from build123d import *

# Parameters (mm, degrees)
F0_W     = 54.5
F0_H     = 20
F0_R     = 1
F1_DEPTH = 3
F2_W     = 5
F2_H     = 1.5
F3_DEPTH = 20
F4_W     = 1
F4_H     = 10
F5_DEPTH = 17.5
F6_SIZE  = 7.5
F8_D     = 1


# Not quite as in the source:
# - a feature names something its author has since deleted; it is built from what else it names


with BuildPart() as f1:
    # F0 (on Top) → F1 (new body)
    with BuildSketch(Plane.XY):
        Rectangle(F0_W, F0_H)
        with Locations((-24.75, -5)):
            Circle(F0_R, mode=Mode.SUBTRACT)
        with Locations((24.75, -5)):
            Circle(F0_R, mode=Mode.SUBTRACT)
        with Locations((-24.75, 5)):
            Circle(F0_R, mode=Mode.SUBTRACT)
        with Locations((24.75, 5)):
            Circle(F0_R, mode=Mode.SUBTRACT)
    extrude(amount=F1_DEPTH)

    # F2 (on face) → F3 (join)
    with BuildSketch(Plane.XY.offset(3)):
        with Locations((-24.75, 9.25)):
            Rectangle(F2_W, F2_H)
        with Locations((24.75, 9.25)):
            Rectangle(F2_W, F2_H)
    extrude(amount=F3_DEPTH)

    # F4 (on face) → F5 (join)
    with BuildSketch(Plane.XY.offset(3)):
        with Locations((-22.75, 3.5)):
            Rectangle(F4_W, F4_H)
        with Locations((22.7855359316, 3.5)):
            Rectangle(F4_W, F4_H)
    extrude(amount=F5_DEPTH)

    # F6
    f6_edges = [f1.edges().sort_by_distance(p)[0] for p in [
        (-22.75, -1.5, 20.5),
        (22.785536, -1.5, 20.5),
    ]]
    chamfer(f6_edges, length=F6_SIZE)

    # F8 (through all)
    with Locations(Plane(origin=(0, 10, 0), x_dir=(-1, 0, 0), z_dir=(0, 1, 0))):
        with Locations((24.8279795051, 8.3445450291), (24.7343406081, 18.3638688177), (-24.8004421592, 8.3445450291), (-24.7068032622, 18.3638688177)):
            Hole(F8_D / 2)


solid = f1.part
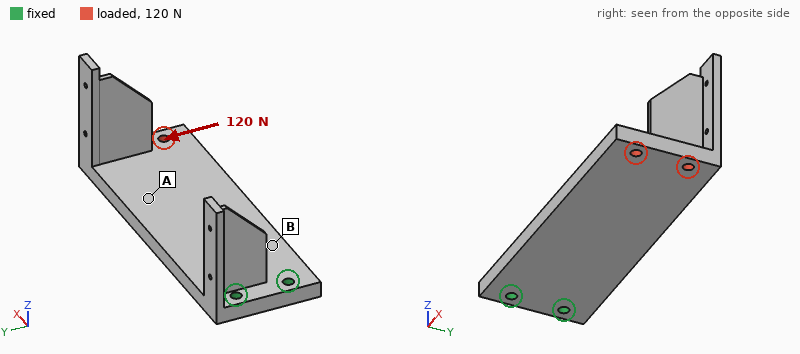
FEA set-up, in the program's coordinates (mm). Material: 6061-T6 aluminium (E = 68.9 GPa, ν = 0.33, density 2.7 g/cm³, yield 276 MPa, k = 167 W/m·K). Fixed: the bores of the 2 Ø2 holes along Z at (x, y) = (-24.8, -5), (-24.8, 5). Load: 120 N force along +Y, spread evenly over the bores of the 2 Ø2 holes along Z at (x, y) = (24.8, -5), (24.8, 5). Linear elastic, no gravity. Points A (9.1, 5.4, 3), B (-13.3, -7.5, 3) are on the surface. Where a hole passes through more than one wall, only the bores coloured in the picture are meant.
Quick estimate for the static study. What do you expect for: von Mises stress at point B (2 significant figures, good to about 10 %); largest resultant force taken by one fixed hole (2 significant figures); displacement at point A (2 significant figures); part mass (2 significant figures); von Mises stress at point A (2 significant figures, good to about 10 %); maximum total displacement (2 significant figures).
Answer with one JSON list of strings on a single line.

["17 MPa", "520 N", "30 µm", "10 g", "6.3 MPa", "55 µm"]
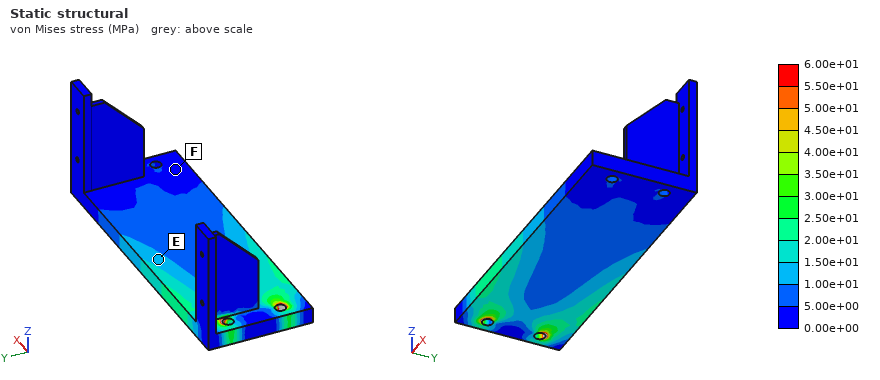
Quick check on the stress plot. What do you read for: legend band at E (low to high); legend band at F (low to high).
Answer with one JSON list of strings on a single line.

["1.00e+01 to 1.50e+01 MPa", "0.00e+00 to 5.00e+00 MPa"]
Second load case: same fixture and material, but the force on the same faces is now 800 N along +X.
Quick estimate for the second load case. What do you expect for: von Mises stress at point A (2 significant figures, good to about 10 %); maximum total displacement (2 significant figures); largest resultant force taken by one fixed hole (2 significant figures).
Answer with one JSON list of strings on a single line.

["13 MPa", "12 µm", "400 N"]
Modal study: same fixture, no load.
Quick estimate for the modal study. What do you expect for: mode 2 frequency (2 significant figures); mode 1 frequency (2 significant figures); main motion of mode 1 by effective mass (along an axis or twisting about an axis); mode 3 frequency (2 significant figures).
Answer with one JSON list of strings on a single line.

["3000 Hz", "780 Hz", "along Z", "3900 Hz"]
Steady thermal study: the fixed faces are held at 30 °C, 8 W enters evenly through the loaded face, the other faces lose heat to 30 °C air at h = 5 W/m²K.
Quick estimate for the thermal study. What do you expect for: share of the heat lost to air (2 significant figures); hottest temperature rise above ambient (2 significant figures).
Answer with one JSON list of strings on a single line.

["4.5 %", "40 K"]
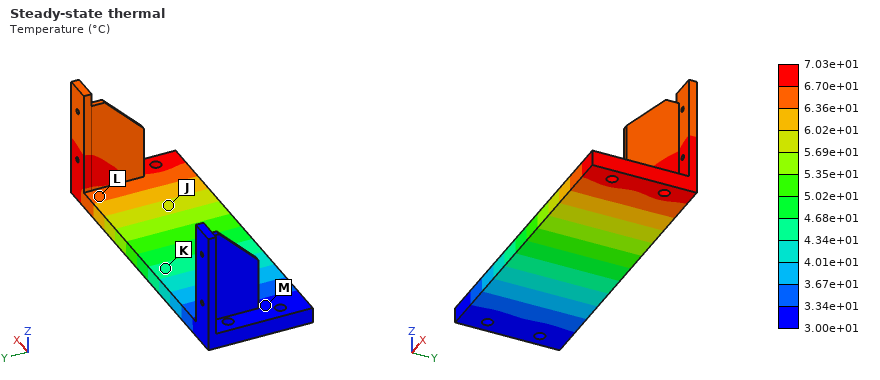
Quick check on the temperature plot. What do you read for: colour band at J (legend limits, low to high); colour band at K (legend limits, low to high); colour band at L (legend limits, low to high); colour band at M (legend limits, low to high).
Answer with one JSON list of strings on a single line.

["5.69e+01 to 6.02e+01 °C", "4.34e+01 to 4.68e+01 °C", "6.36e+01 to 6.70e+01 °C", "3.00e+01 to 3.34e+01 °C"]
